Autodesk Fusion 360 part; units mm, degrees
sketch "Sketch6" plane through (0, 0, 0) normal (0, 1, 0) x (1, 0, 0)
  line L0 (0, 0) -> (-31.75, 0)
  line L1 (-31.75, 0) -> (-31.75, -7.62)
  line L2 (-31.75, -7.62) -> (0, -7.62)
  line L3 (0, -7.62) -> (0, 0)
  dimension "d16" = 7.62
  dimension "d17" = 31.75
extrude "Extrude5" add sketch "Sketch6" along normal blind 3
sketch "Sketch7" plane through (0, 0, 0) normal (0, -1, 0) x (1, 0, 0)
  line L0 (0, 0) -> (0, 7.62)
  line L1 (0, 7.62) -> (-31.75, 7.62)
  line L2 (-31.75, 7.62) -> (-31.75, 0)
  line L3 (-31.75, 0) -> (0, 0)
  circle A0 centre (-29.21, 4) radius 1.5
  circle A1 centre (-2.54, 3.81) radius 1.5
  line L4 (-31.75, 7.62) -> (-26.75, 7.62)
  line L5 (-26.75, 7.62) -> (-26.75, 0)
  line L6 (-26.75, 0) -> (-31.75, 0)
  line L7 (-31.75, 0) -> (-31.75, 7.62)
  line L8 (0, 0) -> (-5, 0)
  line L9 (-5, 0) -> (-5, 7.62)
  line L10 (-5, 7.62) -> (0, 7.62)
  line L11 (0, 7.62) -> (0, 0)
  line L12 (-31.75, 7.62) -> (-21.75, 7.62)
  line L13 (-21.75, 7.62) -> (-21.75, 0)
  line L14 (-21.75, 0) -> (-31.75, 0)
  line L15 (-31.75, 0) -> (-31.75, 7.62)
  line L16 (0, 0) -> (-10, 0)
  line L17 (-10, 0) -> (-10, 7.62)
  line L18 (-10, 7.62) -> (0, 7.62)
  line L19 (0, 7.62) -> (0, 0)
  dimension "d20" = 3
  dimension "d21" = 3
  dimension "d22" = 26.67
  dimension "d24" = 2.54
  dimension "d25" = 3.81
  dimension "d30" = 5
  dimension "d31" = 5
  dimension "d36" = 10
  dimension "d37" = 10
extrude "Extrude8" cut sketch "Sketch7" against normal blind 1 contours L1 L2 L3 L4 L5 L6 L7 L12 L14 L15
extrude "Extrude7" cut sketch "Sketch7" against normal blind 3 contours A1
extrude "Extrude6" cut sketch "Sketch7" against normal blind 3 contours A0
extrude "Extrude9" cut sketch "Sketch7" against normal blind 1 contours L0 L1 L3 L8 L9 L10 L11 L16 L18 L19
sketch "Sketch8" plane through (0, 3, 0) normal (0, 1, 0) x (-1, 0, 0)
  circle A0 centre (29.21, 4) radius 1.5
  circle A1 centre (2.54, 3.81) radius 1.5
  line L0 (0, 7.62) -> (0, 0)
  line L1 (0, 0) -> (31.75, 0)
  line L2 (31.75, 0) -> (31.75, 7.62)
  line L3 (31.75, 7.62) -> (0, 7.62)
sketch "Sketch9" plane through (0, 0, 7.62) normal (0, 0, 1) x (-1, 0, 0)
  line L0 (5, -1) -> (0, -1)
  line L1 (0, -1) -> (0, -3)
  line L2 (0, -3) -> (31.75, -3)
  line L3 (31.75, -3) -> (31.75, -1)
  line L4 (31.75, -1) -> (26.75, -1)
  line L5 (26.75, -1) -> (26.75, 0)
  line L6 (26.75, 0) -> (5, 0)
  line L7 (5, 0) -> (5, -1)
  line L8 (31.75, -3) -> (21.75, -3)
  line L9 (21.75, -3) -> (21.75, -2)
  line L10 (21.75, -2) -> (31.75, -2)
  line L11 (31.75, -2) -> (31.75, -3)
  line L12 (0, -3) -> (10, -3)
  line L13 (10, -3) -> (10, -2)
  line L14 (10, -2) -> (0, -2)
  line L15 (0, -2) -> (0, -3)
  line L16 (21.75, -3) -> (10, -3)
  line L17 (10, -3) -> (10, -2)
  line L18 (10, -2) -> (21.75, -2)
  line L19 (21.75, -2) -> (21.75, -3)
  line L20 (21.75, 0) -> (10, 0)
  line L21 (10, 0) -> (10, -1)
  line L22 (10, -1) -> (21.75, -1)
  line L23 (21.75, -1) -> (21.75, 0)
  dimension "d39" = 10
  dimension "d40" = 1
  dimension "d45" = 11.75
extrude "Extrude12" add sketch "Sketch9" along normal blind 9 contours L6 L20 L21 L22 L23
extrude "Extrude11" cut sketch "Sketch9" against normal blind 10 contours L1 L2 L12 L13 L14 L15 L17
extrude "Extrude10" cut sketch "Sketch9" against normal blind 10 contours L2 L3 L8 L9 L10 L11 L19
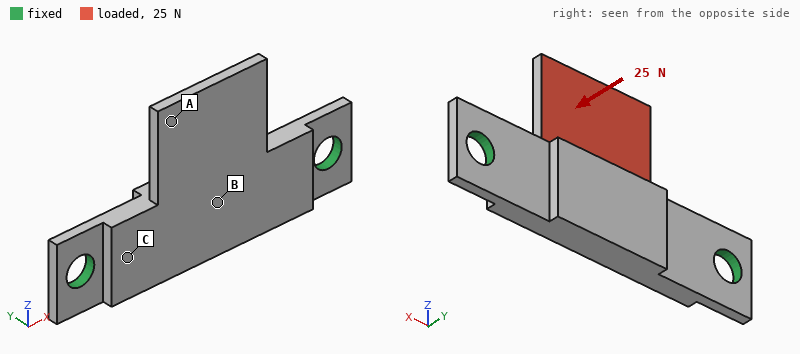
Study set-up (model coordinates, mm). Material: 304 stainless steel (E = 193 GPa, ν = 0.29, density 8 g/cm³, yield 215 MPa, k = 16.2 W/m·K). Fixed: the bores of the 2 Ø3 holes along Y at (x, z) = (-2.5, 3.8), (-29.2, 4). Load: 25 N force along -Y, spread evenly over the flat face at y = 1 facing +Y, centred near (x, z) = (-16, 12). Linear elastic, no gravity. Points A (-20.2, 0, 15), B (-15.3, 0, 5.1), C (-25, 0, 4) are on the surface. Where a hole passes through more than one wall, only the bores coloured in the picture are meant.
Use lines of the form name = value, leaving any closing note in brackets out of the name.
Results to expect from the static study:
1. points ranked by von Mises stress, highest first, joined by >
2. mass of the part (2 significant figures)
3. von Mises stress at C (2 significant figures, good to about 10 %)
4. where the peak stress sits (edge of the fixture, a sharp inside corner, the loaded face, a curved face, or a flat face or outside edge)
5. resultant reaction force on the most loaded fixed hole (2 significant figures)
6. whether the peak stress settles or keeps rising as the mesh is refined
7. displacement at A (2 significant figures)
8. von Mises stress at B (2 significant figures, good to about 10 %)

points ranked by von Mises stress, highest first, joined by > = C > B > A
mass of the part = 4.7 g
von Mises stress at C = 26 MPa
where the peak stress sits = edge of the fixture
resultant reaction force on the most loaded fixed hole = 19 N
whether the peak stress settles or keeps rising as the mesh is refined = keeps rising
displacement at A = 24 µm
von Mises stress at B = 13 MPa
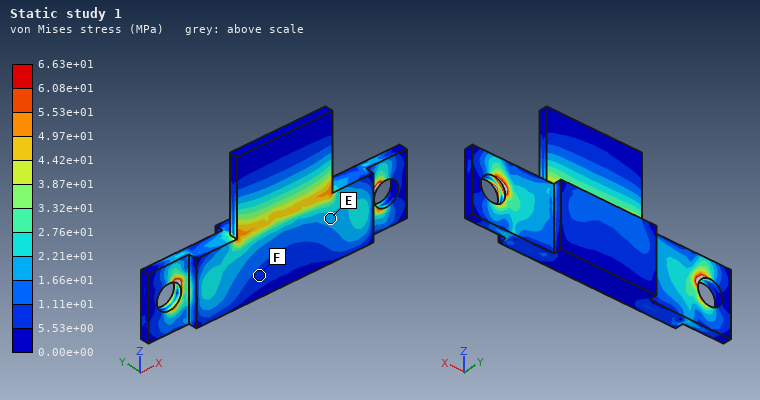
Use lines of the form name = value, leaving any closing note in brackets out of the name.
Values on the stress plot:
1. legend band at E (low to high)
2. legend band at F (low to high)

legend band at E = 1.66e+01 to 2.21e+01 MPa
legend band at F = 5.53e+00 to 1.11e+01 MPa
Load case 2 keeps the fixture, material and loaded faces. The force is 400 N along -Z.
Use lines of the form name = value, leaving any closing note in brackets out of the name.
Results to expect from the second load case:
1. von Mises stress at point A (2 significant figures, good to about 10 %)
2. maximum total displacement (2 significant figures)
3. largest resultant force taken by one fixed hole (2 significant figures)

von Mises stress at point A = 13 MPa
maximum total displacement = 25 µm
largest resultant force taken by one fixed hole = 200 N
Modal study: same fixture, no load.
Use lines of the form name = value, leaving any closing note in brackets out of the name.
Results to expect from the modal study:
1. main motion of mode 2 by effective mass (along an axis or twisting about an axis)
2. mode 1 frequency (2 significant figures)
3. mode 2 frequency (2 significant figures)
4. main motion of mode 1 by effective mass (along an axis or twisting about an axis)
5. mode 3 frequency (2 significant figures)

main motion of mode 2 by effective mass = along Y
mode 1 frequency = 6000 Hz
mode 2 frequency = 12 kHz
main motion of mode 1 by effective mass = along Y
mode 3 frequency = 17 kHz
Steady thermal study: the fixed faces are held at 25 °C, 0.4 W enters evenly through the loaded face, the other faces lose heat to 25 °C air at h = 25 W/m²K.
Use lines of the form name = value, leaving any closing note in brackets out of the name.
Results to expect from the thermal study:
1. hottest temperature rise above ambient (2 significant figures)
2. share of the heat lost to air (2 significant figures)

hottest temperature rise above ambient = 17 K
share of the heat lost to air = 27 %
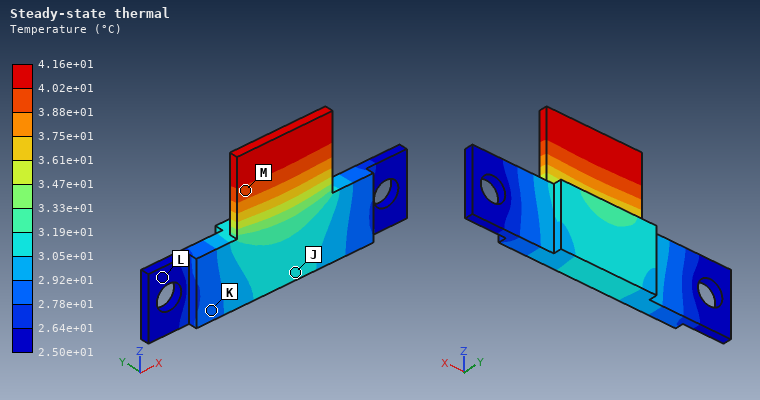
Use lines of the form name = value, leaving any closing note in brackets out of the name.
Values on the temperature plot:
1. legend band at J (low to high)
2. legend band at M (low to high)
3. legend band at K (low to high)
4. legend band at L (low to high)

legend band at J = 3.05e+01 to 3.19e+01 °C
legend band at M = 3.88e+01 to 4.02e+01 °C
legend band at K = 2.78e+01 to 2.92e+01 °C
legend band at L = 2.50e+01 to 2.64e+01 °C
